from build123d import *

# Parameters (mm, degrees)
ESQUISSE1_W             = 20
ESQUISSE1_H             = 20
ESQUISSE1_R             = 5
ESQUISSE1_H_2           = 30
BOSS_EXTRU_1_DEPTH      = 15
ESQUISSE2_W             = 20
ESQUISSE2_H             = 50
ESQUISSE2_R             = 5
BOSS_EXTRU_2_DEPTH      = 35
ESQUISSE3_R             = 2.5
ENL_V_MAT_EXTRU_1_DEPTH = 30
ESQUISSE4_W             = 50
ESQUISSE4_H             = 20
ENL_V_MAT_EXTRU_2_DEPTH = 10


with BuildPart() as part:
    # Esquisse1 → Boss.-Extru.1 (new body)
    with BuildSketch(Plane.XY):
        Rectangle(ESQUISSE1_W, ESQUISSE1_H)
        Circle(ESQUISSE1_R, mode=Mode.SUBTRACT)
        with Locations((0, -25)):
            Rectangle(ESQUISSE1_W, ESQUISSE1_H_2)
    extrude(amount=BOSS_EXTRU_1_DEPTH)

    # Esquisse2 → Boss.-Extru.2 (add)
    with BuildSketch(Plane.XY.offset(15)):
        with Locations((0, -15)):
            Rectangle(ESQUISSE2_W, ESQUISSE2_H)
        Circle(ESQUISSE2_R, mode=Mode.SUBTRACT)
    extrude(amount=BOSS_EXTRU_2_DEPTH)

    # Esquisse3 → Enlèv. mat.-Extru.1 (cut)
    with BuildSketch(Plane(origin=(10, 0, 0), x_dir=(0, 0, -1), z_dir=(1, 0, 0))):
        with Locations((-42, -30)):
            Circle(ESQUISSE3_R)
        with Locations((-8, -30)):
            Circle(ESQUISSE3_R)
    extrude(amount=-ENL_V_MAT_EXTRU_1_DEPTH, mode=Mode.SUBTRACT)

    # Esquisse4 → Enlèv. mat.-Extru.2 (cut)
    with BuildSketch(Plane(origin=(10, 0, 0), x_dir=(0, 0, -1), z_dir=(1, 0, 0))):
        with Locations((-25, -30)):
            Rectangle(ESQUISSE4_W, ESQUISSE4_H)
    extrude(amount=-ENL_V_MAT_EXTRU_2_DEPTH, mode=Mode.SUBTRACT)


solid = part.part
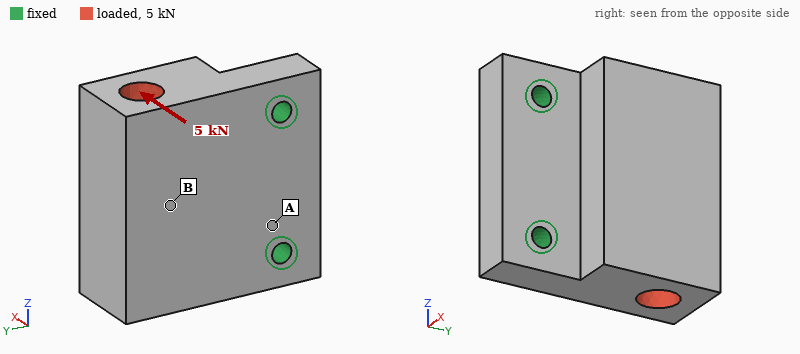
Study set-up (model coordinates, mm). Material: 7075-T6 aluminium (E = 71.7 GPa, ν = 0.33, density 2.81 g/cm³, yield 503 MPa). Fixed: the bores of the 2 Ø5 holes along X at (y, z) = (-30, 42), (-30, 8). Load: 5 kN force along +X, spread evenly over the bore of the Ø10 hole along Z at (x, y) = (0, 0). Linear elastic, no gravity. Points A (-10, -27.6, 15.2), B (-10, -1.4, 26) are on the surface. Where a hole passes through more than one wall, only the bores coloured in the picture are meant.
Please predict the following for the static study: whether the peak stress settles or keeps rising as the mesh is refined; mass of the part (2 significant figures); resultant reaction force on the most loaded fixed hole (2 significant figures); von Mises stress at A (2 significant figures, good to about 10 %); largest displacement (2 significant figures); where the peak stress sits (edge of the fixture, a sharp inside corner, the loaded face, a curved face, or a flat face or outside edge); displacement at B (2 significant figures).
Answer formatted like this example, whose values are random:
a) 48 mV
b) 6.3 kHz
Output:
a) keeps rising
b) 100 g
c) 2.5 kN
d) 95 MPa
e) 0.26 mm
f) edge of the fixture
g) 0.17 mm
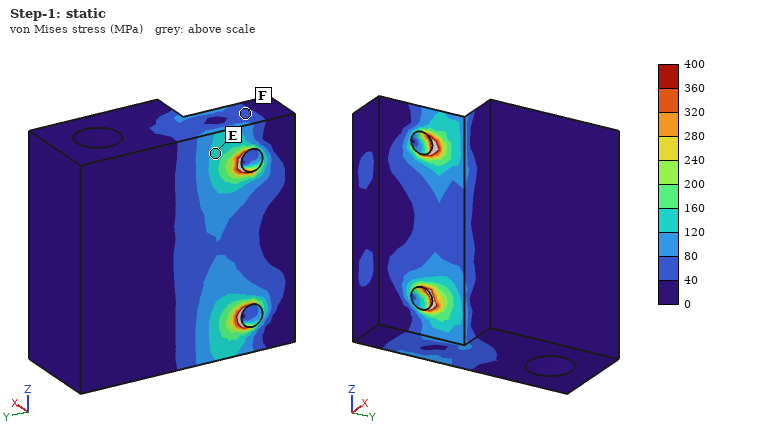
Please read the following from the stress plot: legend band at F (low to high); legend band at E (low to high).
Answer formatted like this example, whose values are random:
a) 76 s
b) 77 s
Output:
a) 40 to 80 MPa
b) 120 to 160 MPa
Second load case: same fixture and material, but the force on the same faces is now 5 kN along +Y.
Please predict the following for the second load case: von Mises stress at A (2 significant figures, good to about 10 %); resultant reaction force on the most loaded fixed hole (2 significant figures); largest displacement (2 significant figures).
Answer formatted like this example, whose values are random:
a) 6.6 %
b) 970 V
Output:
a) 13 MPa
b) 2.5 kN
c) 50 µm
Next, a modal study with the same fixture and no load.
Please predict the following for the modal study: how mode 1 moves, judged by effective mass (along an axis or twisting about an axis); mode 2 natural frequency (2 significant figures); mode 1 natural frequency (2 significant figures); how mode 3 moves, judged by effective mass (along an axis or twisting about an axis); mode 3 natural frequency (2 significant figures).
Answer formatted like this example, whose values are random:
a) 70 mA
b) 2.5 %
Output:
a) along X
b) 10 kHz
c) 3500 Hz
d) along Z
e) 11 kHz
